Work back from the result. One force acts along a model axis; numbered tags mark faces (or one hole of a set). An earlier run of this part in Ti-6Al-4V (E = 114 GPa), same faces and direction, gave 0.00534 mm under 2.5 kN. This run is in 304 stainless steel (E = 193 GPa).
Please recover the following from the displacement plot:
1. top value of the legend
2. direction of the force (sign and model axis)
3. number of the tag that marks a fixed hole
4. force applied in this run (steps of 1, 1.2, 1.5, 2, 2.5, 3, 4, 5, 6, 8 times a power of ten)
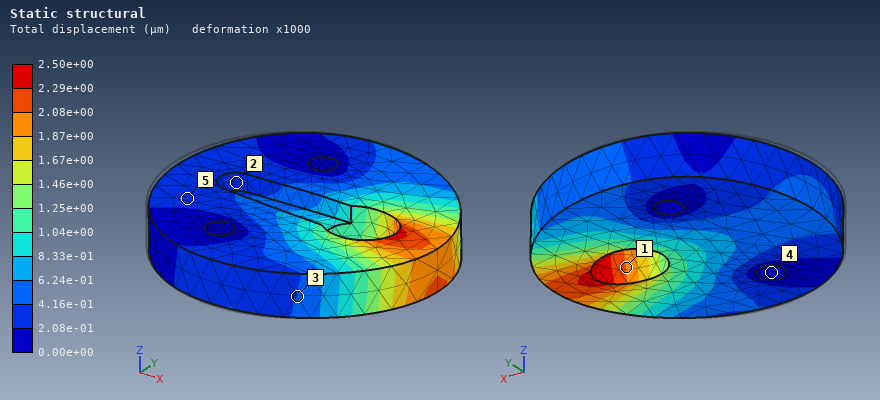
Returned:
2.50e+00 µm
+X
4
2 kN
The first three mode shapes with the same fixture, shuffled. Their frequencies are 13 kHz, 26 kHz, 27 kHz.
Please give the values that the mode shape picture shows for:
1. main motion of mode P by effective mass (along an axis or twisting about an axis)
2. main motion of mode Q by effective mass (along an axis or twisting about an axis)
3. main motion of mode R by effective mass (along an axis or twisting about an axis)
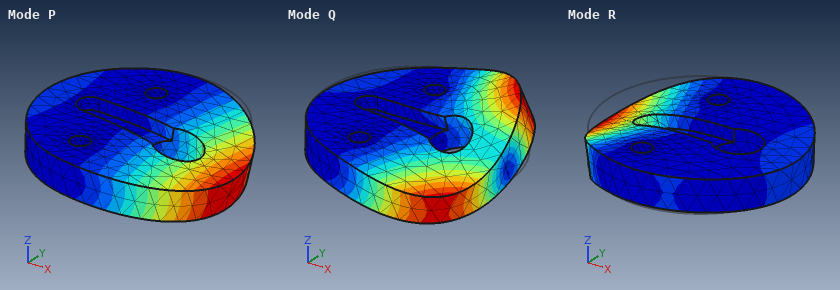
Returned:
along Z
twisting about X
along Z
